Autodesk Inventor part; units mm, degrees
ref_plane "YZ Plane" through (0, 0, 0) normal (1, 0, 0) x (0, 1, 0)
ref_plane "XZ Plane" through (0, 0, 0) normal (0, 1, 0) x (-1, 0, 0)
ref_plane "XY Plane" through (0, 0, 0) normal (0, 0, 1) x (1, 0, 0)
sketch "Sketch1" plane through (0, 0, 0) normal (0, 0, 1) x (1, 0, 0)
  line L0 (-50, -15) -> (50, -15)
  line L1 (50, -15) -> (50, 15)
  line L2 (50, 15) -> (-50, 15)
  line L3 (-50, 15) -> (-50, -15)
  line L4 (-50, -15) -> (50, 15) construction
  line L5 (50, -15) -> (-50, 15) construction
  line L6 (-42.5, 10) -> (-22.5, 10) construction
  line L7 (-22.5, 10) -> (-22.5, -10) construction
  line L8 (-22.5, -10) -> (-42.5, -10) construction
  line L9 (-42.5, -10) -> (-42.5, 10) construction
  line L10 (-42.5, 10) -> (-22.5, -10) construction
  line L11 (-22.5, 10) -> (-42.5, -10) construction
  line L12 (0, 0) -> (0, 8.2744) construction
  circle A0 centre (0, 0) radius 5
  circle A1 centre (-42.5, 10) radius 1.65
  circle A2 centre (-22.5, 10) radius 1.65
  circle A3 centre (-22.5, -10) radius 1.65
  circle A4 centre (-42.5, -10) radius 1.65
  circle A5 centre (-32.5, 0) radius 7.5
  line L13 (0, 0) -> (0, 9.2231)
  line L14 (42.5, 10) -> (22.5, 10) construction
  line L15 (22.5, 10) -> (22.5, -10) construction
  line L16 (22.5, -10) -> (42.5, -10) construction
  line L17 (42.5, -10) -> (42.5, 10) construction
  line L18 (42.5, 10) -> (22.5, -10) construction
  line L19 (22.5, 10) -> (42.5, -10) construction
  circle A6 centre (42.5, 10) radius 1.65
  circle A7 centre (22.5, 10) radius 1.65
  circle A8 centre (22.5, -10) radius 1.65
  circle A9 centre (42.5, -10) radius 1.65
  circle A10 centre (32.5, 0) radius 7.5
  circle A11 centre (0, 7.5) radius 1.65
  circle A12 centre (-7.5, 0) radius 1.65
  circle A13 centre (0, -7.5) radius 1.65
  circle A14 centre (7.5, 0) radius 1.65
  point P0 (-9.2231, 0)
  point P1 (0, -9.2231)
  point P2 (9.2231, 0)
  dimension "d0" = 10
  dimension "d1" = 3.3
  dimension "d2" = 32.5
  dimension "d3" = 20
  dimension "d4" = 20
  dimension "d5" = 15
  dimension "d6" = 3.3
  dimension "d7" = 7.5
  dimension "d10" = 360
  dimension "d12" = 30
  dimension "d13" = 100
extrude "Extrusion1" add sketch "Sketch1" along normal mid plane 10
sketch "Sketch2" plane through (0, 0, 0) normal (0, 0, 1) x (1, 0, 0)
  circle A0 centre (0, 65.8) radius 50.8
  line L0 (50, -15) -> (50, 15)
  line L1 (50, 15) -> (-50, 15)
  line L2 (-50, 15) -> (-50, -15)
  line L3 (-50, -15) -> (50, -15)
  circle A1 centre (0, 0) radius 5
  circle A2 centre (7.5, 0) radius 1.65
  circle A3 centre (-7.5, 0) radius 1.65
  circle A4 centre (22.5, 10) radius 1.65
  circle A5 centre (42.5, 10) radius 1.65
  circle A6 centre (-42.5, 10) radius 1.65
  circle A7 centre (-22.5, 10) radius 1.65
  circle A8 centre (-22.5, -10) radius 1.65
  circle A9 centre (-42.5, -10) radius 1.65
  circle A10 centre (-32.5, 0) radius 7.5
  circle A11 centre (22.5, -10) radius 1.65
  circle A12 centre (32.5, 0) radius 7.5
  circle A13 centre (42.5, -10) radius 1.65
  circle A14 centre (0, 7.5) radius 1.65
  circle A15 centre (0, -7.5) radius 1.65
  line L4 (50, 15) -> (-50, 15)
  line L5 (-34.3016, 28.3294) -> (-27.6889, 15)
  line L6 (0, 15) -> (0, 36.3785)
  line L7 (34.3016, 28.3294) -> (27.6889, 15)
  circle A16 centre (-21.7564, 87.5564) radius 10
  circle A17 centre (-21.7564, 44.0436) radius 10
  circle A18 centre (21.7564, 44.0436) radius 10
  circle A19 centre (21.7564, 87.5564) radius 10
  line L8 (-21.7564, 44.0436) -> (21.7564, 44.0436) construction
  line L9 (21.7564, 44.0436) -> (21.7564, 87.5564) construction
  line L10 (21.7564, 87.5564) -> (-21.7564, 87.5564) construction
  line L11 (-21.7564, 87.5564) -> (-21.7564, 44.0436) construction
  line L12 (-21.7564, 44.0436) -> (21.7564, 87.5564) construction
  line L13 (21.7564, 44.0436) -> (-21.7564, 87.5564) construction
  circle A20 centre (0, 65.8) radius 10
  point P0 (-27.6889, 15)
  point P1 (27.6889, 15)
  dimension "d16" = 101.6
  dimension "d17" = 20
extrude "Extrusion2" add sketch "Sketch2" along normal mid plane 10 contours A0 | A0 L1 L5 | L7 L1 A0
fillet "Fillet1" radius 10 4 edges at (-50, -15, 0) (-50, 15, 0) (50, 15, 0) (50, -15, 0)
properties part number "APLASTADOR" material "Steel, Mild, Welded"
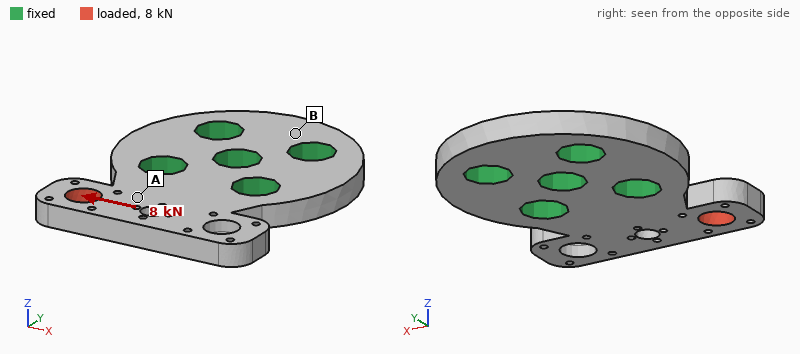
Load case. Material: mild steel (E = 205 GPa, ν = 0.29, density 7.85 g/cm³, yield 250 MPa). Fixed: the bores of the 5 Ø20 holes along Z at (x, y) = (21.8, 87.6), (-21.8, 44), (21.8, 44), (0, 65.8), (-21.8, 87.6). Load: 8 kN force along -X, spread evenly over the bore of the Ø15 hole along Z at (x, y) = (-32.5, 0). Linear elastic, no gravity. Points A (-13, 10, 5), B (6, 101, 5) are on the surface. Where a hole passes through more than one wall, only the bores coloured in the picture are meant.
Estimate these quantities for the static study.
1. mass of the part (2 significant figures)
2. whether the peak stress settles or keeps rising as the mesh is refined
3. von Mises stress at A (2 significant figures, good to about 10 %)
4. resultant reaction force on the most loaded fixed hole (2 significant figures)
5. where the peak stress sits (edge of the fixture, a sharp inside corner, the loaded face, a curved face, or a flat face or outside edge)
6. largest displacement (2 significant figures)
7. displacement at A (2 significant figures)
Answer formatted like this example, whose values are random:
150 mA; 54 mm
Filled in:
720 g; keeps rising; 31 MPa; 6.9 kN; a sharp inside corner; 23 µm; 6.5 µm
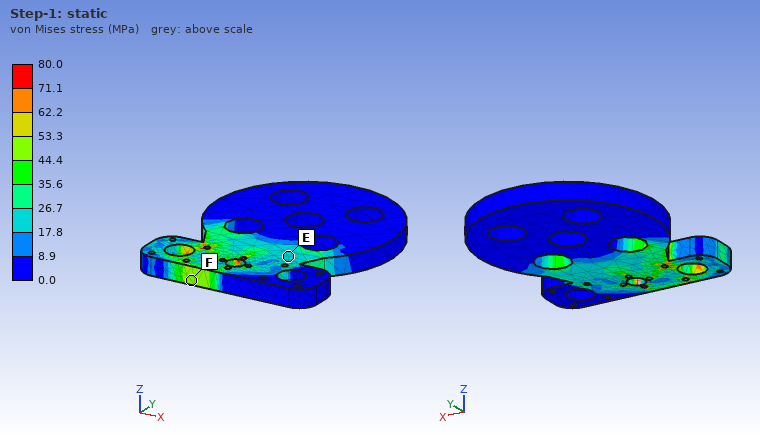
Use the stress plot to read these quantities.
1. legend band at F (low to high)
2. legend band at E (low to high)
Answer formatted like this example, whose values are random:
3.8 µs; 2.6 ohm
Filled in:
44.4 to 53.3 MPa; 17.8 to 26.7 MPa
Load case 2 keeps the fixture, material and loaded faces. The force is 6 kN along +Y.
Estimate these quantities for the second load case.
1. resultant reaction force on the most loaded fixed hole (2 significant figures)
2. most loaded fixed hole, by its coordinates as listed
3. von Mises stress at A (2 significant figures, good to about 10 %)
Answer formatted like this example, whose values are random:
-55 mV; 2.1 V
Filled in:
6.7 kN; (-21.8, 44); 13 MPa
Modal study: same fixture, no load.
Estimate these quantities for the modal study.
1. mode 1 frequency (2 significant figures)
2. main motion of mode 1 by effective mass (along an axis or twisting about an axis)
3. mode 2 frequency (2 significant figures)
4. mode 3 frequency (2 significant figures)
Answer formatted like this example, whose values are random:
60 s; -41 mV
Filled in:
2700 Hz; along Z; 3400 Hz; 6100 Hz
